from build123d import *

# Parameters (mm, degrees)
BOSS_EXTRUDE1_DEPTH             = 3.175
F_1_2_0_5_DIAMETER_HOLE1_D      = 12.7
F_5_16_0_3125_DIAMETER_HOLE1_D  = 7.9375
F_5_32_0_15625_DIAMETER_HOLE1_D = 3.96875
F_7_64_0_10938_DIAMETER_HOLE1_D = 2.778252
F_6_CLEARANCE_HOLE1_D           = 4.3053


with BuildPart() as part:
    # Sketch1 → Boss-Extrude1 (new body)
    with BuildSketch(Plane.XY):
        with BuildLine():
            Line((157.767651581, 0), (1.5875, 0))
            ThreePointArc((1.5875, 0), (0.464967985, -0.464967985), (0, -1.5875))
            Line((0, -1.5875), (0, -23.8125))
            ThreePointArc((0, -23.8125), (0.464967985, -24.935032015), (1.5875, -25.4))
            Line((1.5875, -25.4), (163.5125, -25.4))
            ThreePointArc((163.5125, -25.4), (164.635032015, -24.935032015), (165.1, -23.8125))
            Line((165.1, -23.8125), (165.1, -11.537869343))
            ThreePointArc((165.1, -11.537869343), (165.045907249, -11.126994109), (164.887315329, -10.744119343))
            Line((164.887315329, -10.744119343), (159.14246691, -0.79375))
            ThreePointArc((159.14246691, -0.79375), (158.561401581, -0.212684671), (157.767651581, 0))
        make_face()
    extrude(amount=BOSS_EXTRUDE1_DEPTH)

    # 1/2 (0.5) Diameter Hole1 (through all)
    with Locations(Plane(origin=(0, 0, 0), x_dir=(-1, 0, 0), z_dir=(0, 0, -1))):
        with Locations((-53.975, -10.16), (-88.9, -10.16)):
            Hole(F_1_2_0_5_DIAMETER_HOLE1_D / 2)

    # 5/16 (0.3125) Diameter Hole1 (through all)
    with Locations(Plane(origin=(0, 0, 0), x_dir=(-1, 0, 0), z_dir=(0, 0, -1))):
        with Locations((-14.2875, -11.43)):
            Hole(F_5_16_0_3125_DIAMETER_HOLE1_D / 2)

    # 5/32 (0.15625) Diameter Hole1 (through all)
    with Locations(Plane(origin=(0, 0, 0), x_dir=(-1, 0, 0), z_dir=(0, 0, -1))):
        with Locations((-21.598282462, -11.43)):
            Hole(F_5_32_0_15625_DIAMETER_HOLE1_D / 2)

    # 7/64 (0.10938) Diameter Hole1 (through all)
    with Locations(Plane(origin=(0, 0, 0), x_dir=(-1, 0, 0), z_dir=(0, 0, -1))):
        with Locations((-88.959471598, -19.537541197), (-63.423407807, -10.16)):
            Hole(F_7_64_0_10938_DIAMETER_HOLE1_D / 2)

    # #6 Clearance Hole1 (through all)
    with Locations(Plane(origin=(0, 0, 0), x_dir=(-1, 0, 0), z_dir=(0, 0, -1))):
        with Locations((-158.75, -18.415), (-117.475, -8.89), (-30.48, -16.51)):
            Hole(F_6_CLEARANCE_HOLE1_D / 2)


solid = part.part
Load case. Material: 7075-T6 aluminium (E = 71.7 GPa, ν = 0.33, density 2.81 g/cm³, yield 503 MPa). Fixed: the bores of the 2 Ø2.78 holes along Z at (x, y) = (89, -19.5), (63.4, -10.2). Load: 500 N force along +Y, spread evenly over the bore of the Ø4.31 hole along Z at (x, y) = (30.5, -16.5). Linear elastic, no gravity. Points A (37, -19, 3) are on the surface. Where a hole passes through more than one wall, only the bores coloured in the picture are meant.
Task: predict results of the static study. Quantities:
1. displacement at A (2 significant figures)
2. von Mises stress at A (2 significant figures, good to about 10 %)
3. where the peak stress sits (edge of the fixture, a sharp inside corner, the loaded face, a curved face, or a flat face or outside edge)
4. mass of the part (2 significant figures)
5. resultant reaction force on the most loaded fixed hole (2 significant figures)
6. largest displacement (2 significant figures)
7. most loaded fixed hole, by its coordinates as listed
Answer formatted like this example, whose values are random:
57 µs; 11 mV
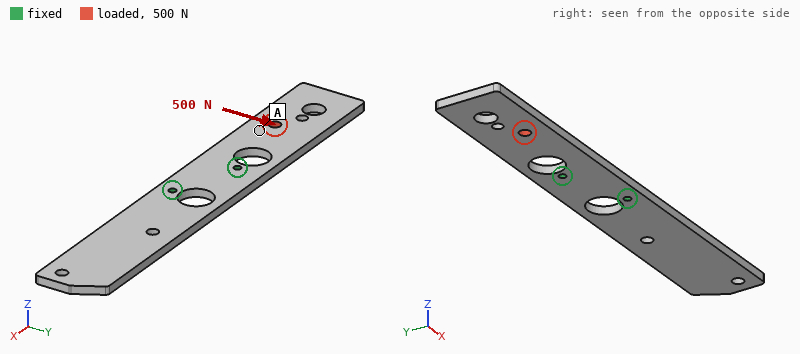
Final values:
0.062 mm; 11 MPa; edge of the fixture; 34 g; 1.0 kN; 0.14 mm; (63.4, -10.2)
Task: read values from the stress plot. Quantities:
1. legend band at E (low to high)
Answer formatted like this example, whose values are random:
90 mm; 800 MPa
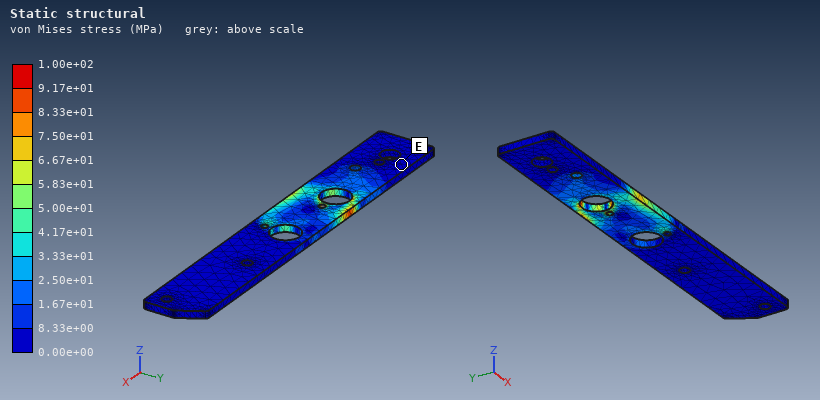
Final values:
0.00e+00 to 8.33e+00 MPa
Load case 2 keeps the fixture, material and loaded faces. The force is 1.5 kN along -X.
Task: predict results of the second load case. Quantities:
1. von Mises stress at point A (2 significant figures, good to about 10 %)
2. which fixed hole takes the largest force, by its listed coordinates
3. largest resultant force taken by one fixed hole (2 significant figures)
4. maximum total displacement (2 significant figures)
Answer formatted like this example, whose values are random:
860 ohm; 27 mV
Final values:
33 MPa; (63.4, -10.2); 870 N; 50 µm
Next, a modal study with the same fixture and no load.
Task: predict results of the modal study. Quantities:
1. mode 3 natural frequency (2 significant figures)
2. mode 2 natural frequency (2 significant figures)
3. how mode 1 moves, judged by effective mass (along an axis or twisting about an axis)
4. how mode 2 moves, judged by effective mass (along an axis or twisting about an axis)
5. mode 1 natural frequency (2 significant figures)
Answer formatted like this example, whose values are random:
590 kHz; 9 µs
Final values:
2100 Hz; 500 Hz; along Z; along Z; 400 Hz
